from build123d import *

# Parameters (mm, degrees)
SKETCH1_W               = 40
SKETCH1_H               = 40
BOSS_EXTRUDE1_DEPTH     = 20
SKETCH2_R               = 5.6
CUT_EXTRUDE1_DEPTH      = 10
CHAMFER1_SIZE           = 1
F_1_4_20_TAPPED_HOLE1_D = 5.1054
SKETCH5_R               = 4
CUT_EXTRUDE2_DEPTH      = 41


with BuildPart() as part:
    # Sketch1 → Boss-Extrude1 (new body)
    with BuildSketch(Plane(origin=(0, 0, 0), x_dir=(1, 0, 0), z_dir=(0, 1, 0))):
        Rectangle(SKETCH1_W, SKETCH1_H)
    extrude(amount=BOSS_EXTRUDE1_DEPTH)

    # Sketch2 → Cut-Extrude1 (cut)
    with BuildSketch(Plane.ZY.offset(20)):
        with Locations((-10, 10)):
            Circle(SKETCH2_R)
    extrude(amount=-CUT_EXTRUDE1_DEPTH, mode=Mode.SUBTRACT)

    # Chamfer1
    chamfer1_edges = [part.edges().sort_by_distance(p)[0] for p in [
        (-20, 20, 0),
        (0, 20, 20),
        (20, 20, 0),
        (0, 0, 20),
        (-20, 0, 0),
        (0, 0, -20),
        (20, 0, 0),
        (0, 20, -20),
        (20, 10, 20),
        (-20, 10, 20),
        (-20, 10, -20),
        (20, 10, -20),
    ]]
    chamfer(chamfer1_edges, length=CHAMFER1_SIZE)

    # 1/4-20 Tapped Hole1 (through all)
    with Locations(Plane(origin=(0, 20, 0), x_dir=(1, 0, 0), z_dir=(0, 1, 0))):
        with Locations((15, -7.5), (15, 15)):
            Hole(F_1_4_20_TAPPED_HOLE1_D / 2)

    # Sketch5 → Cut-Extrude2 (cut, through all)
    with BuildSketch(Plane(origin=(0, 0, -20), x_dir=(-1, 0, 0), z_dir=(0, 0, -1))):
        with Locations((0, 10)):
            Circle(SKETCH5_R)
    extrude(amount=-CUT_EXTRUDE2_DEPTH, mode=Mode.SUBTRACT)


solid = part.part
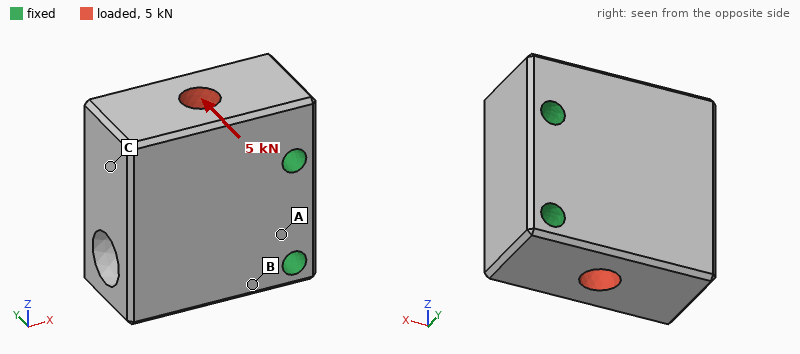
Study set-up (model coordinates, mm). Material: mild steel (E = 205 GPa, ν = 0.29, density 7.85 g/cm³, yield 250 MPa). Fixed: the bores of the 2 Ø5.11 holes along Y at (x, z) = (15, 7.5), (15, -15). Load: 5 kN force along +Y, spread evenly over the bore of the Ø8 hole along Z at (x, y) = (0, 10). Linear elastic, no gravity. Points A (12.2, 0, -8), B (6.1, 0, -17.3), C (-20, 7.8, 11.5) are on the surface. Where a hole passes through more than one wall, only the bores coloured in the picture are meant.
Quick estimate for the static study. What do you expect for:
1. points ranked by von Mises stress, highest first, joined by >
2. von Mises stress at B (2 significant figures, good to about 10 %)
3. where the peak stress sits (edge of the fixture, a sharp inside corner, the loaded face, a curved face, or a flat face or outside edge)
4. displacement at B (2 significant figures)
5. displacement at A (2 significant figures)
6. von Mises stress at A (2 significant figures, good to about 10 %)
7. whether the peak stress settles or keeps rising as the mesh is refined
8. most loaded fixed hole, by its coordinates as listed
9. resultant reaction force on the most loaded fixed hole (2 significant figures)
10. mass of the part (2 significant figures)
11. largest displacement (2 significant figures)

B > A > C
22 MPa
edge of the fixture
1.8 µm
1.2 µm
14 MPa
keeps rising
(15, 7.5)
2.9 kN
220 g
6.9 µm
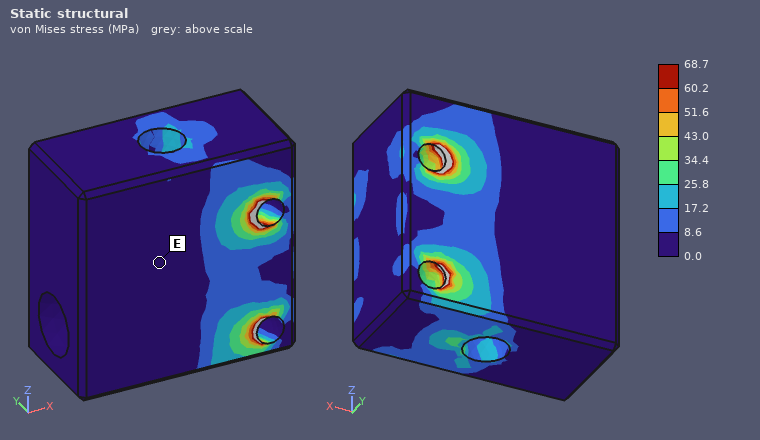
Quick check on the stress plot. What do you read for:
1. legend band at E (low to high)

0.0 to 8.6 MPa
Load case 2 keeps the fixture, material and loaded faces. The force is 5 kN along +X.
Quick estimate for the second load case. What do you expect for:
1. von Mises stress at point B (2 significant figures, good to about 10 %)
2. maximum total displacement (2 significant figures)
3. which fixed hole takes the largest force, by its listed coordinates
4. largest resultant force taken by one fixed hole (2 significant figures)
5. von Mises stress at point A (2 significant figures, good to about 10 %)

5.4 MPa
1.1 µm
(15, 7.5)
3.2 kN
3.6 MPa
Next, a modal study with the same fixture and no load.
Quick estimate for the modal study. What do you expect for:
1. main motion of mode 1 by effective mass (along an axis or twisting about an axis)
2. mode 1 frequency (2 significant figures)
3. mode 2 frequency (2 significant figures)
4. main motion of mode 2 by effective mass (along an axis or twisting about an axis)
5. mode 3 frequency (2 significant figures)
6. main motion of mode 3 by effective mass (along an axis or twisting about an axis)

along Y
9900 Hz
14 kHz
along Z
17 kHz
twisting about X
